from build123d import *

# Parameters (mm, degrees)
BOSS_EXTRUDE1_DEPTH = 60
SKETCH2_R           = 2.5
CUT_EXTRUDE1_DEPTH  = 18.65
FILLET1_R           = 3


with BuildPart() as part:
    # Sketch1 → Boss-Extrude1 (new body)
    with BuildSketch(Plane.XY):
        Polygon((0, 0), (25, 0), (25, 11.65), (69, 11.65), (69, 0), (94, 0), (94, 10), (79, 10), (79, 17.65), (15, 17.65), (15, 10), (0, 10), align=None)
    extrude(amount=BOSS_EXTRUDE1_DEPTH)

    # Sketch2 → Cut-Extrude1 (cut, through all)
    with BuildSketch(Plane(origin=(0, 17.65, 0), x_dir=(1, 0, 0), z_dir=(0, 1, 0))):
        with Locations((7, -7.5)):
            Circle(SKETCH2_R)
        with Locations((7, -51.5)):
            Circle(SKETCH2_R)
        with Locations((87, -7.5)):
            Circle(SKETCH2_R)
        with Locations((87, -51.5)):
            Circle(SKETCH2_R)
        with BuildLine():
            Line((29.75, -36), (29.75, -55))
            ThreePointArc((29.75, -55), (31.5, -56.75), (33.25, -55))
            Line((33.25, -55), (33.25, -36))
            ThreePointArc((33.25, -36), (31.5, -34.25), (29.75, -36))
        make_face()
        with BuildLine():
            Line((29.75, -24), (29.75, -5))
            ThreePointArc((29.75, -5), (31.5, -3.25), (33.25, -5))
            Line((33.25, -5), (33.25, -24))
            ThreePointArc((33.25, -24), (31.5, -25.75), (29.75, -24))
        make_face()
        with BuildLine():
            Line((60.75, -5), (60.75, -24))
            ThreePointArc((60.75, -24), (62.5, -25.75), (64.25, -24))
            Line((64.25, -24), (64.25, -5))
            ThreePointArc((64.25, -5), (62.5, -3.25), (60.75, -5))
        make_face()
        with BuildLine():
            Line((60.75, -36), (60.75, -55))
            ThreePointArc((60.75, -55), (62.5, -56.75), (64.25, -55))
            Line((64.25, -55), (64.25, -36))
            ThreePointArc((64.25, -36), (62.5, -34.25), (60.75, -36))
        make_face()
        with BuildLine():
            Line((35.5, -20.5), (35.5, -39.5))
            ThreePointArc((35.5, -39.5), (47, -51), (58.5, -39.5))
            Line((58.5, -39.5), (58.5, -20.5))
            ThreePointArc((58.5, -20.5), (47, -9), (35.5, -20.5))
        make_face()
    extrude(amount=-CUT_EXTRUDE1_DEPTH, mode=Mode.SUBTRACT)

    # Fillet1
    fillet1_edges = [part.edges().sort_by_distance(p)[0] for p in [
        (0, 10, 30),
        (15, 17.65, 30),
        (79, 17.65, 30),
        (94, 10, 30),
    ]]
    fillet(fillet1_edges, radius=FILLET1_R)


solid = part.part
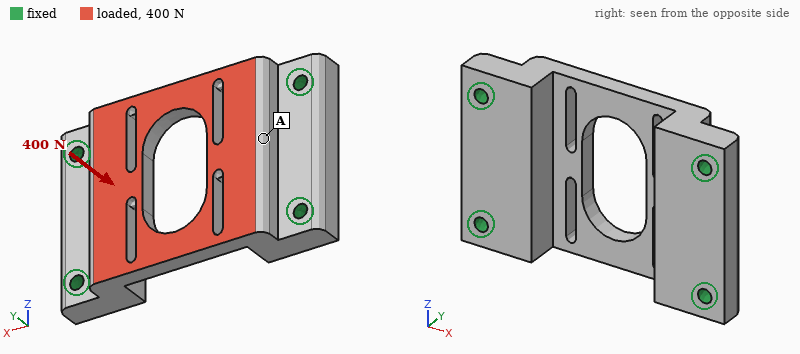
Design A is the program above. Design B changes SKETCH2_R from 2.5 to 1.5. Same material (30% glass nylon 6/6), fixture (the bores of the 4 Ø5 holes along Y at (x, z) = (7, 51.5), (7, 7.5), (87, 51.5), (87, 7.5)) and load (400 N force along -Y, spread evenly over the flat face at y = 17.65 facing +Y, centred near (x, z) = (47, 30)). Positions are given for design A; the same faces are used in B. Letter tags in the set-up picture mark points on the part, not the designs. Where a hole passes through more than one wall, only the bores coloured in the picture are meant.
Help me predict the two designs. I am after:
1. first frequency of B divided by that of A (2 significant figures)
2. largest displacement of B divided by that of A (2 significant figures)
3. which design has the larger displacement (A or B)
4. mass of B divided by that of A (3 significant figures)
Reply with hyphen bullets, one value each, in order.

- 0.92
- 1.1
- B
- 1.01
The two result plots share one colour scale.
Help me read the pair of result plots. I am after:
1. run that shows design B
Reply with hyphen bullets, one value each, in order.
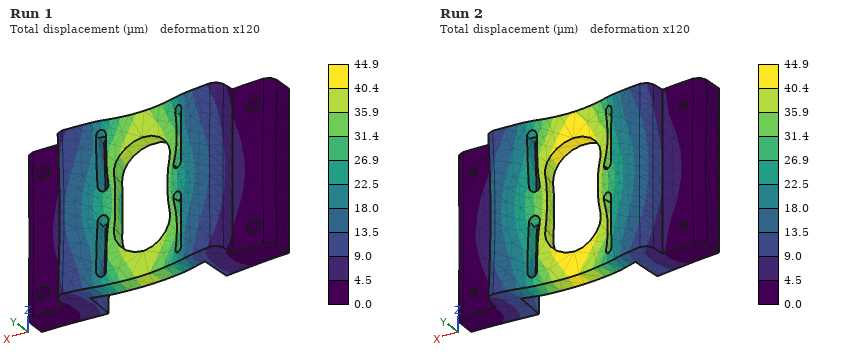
- Run 2
